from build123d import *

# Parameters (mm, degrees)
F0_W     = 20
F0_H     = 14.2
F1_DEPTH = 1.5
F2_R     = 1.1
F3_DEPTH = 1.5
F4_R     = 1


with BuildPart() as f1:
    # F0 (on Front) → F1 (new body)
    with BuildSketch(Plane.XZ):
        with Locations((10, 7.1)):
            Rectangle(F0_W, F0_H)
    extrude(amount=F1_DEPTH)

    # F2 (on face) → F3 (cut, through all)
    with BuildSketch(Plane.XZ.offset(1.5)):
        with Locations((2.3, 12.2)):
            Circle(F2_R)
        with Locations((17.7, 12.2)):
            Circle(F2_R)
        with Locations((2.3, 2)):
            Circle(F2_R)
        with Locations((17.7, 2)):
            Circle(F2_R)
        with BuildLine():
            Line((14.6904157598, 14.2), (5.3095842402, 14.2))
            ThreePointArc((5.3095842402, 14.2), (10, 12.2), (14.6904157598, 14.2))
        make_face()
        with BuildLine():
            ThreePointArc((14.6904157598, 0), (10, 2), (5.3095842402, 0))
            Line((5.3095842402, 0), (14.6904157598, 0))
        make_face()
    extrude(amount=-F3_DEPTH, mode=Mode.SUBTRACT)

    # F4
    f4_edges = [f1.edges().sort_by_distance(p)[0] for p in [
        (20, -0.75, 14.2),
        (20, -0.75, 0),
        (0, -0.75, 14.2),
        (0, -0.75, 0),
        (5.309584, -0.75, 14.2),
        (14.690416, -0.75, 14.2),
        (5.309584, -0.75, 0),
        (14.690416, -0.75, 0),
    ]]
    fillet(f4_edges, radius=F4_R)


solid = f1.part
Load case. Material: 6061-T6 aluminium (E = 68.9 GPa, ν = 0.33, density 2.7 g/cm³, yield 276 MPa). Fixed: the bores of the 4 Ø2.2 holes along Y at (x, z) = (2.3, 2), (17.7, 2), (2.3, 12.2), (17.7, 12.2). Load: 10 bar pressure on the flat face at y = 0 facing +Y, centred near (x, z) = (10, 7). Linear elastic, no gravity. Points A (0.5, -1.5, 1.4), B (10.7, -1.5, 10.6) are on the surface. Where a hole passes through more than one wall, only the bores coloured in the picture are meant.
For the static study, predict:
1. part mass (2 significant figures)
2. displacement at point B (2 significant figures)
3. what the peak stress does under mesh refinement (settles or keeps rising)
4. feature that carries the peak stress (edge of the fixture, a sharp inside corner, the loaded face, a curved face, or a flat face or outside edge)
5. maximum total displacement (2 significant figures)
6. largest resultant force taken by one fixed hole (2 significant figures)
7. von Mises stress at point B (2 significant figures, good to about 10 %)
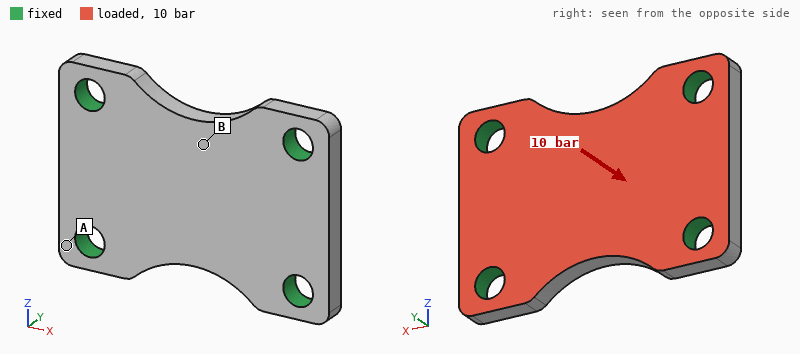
0.98 g
6.6 µm
keeps rising
edge of the fixture
7.4 µm
61 N
22 MPa
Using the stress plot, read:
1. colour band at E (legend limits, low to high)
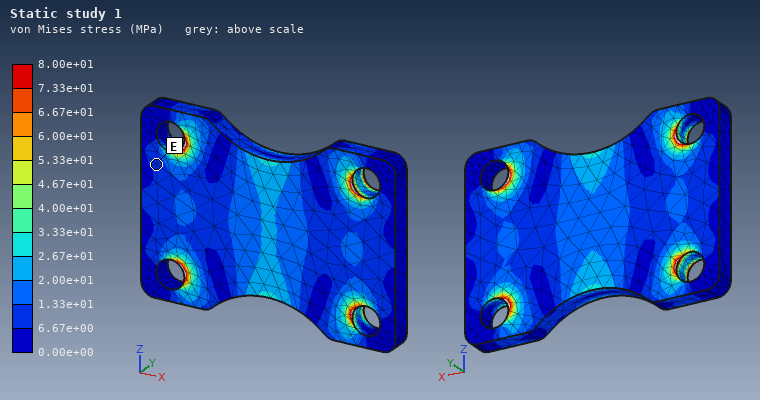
6.67e+00 to 1.33e+01 MPa
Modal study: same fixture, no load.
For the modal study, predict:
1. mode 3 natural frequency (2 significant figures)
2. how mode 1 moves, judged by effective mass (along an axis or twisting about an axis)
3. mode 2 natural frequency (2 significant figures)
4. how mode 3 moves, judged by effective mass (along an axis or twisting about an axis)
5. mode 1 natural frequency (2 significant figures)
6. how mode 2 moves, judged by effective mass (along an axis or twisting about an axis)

75 kHz
along Y
55 kHz
twisting about Z
34 kHz
twisting about X
